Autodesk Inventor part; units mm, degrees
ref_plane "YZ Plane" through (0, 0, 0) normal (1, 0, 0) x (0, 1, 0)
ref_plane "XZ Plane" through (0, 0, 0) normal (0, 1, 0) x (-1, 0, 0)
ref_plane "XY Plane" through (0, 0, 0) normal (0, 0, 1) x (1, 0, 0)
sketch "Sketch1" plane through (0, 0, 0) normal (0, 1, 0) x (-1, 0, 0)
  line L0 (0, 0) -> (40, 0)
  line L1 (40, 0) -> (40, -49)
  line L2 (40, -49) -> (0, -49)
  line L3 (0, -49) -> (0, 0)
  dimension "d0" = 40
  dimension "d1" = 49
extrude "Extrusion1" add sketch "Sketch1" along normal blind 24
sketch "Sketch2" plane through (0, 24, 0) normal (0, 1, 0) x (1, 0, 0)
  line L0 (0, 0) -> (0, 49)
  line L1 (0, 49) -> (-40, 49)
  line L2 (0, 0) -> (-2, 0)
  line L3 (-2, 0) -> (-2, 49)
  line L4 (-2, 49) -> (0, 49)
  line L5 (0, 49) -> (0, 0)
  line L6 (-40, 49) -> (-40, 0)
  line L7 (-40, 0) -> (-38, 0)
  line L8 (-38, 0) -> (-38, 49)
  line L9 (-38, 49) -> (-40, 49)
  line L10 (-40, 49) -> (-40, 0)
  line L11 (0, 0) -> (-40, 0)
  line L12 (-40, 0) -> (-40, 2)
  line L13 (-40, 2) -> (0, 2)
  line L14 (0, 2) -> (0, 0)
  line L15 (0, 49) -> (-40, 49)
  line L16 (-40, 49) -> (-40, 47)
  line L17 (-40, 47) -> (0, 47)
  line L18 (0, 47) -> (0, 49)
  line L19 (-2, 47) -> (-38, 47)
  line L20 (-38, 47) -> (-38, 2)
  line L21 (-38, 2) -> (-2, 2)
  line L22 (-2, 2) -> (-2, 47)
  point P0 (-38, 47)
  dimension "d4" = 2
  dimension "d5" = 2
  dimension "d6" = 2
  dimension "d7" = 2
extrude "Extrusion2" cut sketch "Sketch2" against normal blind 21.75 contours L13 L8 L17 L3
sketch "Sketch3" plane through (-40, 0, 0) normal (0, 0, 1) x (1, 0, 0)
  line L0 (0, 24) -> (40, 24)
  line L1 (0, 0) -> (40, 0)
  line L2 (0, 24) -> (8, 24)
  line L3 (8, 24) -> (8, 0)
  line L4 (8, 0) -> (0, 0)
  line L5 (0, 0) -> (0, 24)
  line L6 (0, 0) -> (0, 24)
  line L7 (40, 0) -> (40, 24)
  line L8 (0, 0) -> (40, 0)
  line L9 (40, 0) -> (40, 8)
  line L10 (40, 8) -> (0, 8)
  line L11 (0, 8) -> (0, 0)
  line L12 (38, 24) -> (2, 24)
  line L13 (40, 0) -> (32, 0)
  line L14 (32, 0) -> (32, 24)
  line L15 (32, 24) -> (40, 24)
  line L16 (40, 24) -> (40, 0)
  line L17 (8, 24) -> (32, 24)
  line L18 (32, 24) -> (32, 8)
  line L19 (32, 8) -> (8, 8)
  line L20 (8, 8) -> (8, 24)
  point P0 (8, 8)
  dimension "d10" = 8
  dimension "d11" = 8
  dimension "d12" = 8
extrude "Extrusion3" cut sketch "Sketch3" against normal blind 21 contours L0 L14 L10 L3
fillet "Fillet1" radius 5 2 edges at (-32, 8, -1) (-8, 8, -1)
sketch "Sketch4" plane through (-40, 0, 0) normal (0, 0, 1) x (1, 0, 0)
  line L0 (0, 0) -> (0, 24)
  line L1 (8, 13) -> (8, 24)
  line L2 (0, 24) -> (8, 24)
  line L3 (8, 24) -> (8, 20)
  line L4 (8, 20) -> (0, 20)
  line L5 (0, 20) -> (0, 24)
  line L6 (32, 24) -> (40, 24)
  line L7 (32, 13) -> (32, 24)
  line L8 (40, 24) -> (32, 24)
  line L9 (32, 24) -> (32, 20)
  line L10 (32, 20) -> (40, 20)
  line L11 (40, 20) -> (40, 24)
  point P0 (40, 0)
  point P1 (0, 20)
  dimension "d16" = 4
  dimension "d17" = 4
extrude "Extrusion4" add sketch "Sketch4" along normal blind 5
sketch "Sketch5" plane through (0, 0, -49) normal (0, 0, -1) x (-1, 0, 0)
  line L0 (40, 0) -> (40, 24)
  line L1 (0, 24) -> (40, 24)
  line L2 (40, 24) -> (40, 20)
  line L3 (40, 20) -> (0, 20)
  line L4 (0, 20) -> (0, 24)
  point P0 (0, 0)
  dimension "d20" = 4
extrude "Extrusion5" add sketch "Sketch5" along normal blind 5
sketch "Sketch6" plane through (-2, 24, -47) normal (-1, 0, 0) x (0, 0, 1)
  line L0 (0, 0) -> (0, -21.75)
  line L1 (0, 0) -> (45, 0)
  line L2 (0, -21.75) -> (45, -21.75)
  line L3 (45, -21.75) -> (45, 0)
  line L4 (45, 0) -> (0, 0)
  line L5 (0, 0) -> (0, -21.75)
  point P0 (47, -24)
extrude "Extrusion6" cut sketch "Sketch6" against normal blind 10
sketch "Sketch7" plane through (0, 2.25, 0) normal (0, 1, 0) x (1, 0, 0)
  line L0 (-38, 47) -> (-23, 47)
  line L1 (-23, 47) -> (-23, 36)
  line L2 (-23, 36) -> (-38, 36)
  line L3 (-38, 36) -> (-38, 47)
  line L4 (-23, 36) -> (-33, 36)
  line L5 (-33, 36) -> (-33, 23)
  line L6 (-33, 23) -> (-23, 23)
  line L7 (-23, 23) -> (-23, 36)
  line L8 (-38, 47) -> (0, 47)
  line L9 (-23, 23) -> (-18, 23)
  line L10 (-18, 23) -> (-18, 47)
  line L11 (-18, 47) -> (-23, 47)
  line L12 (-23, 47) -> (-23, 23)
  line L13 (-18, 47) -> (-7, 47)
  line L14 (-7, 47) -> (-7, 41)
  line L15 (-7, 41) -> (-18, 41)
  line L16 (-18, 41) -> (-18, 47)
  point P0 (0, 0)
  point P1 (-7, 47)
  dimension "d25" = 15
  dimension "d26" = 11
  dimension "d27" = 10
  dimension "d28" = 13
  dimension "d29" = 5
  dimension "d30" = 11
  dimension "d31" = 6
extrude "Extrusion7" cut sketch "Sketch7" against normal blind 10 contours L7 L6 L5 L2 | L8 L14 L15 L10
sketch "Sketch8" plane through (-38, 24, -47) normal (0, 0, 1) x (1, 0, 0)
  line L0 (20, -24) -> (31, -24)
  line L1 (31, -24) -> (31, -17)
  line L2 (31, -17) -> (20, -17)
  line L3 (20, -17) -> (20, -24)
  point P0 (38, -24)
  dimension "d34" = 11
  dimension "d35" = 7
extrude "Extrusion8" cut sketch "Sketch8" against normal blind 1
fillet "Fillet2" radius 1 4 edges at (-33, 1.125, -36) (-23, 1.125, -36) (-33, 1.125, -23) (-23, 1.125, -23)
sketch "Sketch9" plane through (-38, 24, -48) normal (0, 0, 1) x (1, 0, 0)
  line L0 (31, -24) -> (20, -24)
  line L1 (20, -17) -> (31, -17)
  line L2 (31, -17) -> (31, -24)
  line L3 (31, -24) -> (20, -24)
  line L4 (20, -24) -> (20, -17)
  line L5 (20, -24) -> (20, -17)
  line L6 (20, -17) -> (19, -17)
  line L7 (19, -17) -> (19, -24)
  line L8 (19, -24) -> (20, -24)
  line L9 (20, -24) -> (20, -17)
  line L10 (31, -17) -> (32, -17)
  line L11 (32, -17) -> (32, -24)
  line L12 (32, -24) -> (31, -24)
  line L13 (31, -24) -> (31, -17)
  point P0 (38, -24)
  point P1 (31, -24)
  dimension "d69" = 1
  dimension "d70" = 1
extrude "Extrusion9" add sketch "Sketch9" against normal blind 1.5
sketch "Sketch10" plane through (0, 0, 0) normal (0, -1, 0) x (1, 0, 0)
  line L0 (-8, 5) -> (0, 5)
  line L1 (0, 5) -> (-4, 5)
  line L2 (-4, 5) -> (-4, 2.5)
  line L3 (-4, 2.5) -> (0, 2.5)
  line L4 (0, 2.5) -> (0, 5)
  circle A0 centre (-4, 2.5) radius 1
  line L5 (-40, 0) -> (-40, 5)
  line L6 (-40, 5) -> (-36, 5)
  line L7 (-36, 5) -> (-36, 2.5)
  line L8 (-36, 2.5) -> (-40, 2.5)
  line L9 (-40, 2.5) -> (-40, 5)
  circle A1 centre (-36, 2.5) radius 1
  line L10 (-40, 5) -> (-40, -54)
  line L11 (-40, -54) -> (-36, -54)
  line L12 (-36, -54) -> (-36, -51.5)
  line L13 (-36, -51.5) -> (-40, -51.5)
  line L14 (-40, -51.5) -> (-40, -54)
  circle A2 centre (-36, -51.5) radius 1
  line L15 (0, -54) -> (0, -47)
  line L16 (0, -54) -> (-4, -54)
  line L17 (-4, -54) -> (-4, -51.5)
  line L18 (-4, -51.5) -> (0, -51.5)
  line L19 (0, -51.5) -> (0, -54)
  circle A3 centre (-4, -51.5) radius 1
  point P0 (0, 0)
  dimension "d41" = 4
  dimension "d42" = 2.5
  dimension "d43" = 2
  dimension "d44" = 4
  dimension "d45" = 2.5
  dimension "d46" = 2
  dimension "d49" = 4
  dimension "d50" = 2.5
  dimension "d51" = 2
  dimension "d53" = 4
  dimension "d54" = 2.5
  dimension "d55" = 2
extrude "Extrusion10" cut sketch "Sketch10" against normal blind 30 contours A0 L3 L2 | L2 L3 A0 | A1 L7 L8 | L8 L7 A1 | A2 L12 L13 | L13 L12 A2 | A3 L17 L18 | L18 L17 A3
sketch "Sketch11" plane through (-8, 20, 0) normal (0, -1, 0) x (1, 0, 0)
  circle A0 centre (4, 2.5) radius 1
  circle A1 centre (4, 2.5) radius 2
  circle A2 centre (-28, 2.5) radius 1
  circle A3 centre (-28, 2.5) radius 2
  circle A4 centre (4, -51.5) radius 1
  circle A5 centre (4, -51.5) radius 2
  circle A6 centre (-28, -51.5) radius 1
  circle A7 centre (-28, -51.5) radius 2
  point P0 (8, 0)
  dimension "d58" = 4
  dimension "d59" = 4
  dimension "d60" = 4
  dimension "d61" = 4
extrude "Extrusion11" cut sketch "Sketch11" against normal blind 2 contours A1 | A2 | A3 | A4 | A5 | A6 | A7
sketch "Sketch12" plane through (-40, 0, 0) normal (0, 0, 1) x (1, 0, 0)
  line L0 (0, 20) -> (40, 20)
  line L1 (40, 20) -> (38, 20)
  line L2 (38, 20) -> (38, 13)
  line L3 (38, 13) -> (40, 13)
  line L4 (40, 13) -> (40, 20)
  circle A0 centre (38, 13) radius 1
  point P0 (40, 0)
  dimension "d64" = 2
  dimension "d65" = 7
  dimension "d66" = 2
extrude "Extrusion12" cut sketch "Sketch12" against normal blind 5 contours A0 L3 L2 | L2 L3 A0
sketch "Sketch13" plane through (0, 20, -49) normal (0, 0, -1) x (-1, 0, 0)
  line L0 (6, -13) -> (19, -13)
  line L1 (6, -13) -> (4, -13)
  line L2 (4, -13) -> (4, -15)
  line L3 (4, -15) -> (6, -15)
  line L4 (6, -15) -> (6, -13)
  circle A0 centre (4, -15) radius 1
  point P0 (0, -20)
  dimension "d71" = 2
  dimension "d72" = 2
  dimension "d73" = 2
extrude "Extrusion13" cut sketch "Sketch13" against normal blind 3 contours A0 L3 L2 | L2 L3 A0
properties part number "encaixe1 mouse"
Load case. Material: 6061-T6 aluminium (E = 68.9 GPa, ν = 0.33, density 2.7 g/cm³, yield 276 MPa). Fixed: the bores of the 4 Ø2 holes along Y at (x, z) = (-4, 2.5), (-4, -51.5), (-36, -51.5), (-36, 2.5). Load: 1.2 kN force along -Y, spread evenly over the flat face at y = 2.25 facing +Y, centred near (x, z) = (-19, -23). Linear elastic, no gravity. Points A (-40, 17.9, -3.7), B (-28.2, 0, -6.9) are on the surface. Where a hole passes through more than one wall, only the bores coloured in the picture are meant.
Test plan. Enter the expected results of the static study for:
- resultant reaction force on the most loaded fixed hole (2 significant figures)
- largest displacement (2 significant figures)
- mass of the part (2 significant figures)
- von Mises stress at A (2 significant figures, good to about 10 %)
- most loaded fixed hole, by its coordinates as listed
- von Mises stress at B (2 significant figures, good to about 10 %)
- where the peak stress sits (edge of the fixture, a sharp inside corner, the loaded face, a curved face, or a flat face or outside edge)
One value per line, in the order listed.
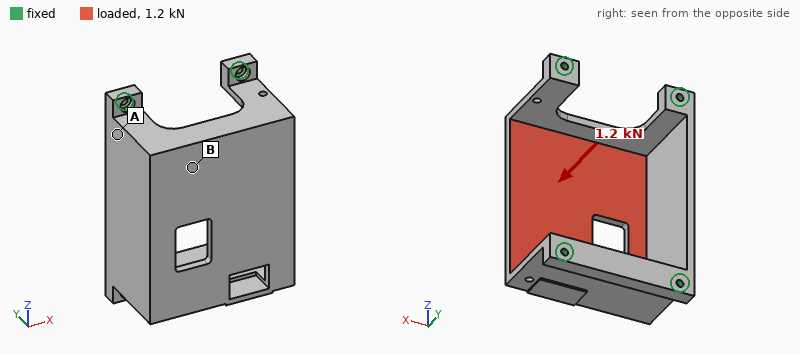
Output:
380 N
0.32 mm
26 g
21 MPa
(-4, 2.5)
56 MPa
a curved face
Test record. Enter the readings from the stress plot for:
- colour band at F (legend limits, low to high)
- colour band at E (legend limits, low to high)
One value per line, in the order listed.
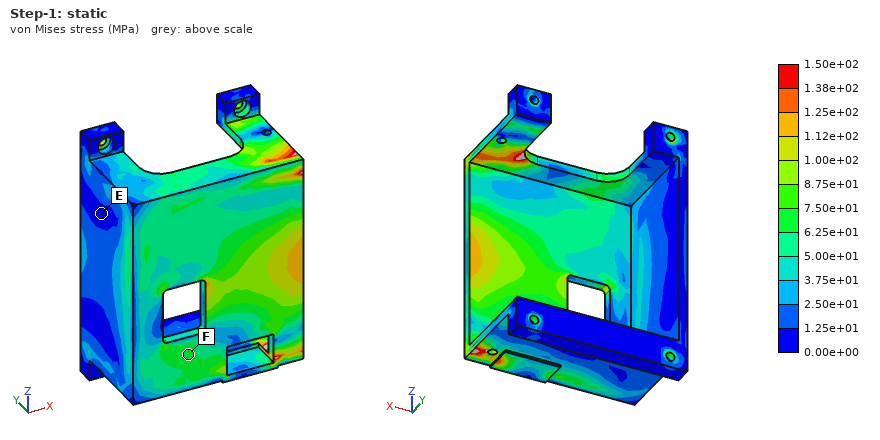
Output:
6.25e+01 to 7.50e+01 MPa
0.00e+00 to 1.25e+01 MPa
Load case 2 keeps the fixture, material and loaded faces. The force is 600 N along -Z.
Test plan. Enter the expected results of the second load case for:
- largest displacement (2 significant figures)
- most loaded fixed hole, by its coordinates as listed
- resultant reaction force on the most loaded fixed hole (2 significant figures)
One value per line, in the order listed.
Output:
77 µm
(-36, -51.5)
510 N
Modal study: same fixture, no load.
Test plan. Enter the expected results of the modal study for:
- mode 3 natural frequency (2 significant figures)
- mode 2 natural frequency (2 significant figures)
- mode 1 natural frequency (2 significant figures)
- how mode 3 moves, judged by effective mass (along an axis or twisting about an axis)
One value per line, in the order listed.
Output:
5800 Hz
4200 Hz
4100 Hz
along X
